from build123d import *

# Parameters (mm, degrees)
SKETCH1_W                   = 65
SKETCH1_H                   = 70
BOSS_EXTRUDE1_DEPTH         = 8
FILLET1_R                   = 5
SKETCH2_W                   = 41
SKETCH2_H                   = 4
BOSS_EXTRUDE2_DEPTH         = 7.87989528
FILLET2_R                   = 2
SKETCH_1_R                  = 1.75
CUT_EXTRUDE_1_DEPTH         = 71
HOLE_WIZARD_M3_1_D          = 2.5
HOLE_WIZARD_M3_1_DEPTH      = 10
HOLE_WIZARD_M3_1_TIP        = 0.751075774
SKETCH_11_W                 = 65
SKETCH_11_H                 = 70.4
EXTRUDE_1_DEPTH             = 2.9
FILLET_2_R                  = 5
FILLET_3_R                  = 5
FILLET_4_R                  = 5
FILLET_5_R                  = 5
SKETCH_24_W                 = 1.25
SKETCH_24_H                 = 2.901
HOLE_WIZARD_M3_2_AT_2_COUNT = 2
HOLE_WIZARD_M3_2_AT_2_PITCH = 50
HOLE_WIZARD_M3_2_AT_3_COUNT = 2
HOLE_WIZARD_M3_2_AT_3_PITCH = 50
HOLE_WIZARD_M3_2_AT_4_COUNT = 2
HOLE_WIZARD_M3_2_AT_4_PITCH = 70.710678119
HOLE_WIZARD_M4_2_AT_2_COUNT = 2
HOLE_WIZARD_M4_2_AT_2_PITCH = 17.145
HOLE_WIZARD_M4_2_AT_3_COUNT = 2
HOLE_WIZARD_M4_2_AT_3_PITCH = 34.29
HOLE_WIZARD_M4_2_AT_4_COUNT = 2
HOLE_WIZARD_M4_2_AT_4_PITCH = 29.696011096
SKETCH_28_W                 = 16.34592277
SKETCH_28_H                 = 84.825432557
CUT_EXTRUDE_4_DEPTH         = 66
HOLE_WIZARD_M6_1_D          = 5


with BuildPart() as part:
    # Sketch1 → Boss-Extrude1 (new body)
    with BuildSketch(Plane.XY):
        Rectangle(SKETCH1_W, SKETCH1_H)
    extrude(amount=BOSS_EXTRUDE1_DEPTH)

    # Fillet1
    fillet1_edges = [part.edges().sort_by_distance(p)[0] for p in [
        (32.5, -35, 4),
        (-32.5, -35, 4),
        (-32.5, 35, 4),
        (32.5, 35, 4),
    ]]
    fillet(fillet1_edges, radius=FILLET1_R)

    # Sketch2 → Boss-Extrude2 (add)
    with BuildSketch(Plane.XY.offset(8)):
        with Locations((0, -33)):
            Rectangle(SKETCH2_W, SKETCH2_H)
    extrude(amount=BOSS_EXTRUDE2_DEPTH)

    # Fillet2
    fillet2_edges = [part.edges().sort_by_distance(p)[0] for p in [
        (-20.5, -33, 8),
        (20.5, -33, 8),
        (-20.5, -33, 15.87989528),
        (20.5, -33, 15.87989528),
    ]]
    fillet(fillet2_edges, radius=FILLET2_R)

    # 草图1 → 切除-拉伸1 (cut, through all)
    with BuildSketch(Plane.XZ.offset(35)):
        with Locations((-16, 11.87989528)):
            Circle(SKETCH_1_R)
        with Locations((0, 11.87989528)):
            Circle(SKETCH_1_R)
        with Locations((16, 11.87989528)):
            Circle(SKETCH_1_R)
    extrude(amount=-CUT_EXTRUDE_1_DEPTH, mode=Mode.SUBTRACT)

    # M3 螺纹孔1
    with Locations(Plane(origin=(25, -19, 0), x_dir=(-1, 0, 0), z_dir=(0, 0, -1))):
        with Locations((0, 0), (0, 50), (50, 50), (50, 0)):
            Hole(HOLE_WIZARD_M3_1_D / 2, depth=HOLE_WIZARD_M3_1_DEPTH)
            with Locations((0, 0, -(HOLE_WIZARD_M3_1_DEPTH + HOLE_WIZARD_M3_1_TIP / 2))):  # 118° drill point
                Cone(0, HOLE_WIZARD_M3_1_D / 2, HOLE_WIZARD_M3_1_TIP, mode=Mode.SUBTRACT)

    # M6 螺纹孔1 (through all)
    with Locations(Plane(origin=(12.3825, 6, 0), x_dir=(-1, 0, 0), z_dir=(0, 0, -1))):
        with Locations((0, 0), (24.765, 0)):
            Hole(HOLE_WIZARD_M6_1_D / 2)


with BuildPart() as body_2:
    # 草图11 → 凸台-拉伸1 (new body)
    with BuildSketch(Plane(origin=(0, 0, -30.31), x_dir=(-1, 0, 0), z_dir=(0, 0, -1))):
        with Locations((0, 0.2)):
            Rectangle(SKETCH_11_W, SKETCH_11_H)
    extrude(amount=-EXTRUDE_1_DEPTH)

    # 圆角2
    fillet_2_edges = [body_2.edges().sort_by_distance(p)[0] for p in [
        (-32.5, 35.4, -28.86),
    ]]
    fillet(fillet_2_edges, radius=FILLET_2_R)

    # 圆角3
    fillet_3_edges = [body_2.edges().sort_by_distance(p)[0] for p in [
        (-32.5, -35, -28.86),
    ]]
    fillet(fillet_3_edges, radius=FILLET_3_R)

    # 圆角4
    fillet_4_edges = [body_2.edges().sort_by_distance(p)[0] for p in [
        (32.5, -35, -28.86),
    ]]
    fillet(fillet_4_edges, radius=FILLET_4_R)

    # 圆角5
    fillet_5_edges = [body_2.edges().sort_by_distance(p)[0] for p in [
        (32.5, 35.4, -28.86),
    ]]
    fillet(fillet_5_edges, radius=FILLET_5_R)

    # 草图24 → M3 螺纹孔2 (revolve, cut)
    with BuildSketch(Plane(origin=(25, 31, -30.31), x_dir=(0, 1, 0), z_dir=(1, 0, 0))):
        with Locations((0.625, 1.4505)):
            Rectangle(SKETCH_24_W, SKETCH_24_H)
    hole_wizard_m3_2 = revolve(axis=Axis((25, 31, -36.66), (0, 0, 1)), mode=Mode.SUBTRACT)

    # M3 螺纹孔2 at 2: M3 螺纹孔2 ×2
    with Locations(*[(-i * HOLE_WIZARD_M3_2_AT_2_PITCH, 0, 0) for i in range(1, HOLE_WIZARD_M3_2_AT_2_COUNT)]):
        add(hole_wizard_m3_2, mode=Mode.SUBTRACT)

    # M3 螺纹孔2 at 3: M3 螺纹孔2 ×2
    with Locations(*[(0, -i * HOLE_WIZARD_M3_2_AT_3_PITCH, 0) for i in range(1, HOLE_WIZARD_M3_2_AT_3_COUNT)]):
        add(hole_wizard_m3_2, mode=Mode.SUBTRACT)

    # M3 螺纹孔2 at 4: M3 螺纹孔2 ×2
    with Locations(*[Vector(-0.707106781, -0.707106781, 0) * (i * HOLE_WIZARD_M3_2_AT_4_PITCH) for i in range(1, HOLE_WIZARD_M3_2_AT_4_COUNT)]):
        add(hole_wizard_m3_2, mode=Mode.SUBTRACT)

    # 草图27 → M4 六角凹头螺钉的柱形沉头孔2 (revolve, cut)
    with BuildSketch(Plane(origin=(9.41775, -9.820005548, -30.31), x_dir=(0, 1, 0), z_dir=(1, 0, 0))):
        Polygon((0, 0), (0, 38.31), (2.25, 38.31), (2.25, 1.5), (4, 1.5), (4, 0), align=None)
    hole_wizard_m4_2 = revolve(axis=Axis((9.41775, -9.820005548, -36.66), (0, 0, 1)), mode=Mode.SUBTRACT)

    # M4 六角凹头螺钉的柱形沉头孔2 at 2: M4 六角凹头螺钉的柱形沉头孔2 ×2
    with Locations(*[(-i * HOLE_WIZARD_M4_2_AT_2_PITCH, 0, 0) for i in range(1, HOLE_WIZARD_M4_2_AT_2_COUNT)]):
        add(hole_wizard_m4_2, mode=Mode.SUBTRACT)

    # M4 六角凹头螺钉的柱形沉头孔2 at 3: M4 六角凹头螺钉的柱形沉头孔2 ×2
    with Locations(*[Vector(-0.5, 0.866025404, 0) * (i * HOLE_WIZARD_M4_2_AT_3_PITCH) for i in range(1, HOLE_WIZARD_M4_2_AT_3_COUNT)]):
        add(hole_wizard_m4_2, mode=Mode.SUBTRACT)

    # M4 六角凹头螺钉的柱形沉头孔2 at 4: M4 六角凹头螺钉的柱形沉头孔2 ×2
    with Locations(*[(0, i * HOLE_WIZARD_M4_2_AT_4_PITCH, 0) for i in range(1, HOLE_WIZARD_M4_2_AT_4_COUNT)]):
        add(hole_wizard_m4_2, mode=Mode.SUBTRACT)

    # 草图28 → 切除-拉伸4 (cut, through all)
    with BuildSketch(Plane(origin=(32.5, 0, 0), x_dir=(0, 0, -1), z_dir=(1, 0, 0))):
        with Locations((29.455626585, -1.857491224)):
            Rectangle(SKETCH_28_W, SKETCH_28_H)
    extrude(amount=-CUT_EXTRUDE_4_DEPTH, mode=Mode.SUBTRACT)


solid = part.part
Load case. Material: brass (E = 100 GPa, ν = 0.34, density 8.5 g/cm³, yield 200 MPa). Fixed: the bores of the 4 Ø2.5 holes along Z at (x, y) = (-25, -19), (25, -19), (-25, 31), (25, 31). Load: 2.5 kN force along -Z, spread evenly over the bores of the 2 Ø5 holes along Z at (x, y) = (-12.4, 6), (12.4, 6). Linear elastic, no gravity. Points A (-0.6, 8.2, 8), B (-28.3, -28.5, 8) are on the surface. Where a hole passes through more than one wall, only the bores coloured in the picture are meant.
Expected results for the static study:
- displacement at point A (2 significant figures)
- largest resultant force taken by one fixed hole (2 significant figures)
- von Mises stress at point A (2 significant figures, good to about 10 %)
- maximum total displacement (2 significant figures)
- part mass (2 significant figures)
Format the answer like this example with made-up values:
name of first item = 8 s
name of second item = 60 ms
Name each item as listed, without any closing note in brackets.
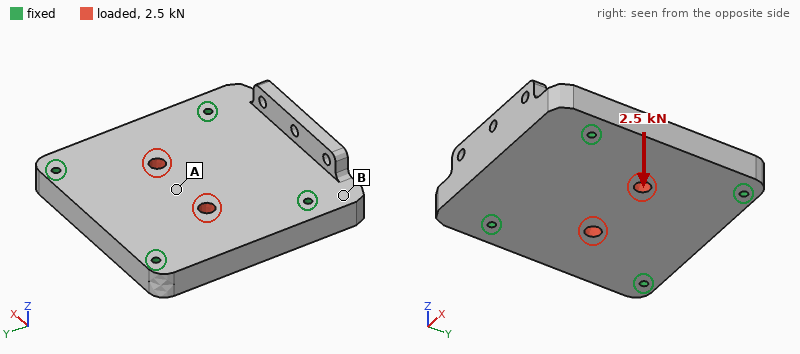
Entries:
displacement at point A = 19 µm
largest resultant force taken by one fixed hole = 630 N
von Mises stress at point A = 26 MPa
maximum total displacement = 20 µm
part mass = 310 g
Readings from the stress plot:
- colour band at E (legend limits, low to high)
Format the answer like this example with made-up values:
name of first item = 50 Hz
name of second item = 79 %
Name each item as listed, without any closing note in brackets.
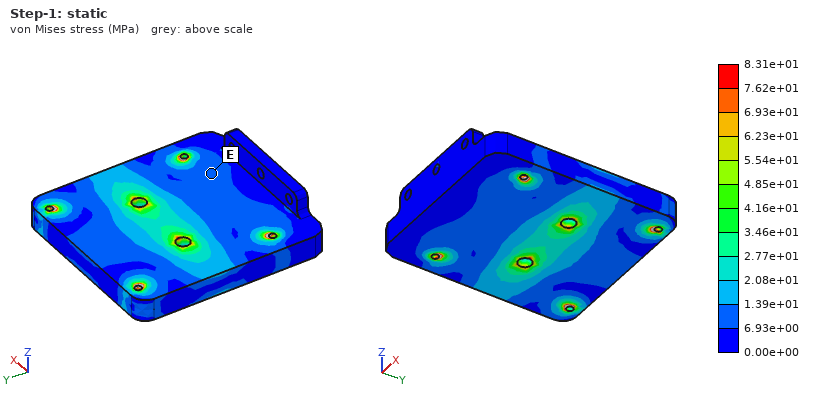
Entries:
colour band at E = 6.93e+00 to 1.39e+01 MPa
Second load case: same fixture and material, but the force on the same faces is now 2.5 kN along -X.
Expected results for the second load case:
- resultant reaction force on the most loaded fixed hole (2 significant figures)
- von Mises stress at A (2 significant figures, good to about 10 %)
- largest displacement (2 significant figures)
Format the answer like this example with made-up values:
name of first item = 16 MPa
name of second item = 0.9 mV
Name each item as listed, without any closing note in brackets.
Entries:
resultant reaction force on the most loaded fixed hole = 710 N
von Mises stress at A = 2.5 MPa
largest displacement = 2.7 µm
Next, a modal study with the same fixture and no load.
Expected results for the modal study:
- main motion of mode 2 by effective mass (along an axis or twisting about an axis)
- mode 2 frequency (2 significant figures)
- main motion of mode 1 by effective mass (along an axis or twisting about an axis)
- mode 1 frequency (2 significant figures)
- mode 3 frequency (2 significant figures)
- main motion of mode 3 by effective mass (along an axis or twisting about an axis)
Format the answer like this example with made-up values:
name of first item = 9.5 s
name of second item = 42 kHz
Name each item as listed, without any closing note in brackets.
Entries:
main motion of mode 2 by effective mass = along Z
mode 2 frequency = 6700 Hz
main motion of mode 1 by effective mass = along Z
mode 1 frequency = 6100 Hz
mode 3 frequency = 9400 Hz
main motion of mode 3 by effective mass = twisting about Y
